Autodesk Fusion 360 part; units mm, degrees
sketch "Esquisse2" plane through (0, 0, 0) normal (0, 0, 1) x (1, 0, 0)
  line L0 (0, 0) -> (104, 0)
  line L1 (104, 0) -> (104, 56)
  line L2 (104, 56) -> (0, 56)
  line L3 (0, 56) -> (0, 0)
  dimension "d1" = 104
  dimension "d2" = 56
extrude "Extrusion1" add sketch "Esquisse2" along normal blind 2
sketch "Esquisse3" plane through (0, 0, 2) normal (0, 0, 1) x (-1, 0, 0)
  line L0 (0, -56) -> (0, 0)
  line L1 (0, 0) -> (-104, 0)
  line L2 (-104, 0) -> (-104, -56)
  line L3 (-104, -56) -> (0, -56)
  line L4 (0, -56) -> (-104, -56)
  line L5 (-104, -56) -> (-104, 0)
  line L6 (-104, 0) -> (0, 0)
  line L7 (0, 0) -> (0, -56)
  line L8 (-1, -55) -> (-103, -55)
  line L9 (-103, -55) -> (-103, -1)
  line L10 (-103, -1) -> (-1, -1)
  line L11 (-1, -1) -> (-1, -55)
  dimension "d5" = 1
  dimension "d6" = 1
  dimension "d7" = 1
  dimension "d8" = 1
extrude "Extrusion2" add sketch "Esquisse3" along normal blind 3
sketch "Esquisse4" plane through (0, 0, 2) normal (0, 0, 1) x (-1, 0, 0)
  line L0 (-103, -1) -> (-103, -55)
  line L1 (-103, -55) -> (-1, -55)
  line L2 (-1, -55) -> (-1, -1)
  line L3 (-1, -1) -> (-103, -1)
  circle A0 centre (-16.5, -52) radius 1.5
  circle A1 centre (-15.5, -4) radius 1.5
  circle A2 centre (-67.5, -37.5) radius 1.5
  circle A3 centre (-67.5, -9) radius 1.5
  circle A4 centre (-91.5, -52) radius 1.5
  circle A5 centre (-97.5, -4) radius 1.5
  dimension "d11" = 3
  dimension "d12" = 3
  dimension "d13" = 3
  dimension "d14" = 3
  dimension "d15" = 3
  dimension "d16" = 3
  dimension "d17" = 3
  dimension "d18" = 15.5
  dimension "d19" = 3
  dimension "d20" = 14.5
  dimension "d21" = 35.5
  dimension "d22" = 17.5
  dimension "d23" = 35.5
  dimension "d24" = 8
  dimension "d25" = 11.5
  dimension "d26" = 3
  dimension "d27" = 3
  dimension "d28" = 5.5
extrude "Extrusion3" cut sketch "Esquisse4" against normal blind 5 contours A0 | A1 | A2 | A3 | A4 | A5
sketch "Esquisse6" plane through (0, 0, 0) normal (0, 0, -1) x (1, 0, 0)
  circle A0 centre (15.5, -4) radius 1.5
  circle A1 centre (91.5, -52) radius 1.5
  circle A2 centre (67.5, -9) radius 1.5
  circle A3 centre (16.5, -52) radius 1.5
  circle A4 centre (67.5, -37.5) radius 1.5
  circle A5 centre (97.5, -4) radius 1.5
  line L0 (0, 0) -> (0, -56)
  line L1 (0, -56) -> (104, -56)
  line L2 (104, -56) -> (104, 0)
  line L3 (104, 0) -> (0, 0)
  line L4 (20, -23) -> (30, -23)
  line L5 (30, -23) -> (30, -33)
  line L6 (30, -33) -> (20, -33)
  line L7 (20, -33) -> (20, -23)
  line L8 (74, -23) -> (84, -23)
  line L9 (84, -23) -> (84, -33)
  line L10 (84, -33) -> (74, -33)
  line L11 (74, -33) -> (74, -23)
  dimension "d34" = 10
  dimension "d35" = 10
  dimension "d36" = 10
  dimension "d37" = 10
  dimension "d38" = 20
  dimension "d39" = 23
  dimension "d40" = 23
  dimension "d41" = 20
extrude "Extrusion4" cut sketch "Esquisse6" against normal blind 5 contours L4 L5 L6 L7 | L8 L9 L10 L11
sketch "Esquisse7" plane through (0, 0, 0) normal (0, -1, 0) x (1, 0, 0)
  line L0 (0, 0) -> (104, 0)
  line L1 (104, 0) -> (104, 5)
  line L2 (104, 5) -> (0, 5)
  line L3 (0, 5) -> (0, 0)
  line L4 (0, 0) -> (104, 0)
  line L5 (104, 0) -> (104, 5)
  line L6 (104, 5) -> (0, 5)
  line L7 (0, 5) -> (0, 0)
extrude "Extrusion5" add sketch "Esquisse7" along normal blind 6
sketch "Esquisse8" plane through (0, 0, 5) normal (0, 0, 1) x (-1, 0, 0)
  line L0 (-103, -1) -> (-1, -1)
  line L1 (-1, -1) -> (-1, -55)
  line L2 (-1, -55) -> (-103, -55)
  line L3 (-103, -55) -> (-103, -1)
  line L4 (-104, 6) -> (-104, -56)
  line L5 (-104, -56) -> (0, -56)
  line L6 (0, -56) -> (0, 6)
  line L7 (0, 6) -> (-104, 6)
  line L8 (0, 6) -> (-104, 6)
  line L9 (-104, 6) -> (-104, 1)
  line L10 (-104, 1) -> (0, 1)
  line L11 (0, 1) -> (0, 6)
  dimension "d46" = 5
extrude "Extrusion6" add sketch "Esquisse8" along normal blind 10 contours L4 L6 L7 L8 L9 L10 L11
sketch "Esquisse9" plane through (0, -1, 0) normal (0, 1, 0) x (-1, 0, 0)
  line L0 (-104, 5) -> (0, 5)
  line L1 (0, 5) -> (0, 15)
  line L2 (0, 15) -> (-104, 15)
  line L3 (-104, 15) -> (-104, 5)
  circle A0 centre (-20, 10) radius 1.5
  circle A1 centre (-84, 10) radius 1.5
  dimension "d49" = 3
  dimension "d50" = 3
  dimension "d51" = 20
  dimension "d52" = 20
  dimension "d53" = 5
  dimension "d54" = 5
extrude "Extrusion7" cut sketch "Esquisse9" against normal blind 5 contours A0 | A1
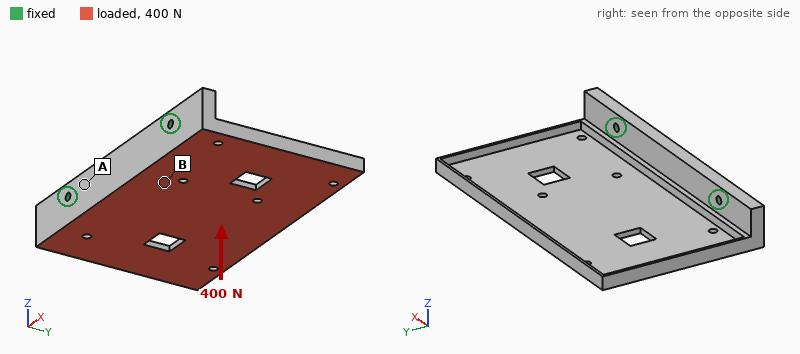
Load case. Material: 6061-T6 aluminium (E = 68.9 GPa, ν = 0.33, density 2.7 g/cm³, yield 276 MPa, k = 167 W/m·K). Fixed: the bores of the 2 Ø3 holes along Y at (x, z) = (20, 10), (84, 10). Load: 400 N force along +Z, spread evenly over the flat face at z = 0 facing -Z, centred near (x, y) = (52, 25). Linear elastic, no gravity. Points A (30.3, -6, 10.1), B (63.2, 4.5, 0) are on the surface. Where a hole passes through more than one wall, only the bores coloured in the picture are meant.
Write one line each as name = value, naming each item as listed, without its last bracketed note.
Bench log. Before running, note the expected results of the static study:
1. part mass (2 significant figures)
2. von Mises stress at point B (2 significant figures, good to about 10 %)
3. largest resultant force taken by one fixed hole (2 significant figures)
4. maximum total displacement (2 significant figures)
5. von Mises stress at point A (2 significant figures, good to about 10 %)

part mass = 55 g
von Mises stress at point B = 83 MPa
largest resultant force taken by one fixed hole = 200 N
maximum total displacement = 1.4 mm
von Mises stress at point A = 26 MPa
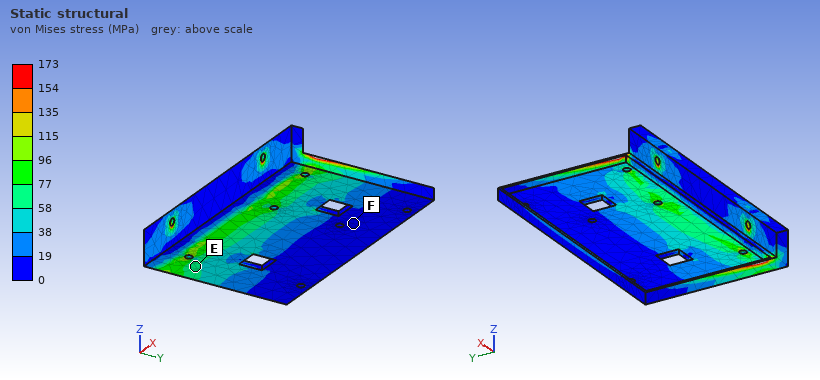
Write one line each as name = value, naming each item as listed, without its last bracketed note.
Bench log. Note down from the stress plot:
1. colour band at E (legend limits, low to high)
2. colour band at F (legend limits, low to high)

colour band at E = 58 to 77 MPa
colour band at F = 0 to 19 MPa
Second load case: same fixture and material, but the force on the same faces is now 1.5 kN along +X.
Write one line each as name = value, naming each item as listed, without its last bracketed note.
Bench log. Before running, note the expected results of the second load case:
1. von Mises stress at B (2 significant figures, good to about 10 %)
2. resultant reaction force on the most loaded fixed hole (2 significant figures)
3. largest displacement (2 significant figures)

von Mises stress at B = 11 MPa
resultant reaction force on the most loaded fixed hole = 1.0 kN
largest displacement = 56 µm
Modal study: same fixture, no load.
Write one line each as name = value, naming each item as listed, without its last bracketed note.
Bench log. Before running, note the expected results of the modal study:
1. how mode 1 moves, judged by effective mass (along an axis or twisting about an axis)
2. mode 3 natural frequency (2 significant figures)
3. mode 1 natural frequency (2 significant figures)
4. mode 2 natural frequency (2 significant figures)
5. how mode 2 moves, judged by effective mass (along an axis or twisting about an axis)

how mode 1 moves, judged by effective mass = along Z
mode 3 natural frequency = 2000 Hz
mode 1 natural frequency = 550 Hz
mode 2 natural frequency = 900 Hz
how mode 2 moves, judged by effective mass = twisting about Y
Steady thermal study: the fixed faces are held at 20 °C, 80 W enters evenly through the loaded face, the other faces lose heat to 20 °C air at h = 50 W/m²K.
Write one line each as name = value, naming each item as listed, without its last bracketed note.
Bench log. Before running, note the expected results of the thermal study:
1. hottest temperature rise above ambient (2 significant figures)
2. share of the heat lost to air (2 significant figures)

hottest temperature rise above ambient = 62 K
share of the heat lost to air = 26 %
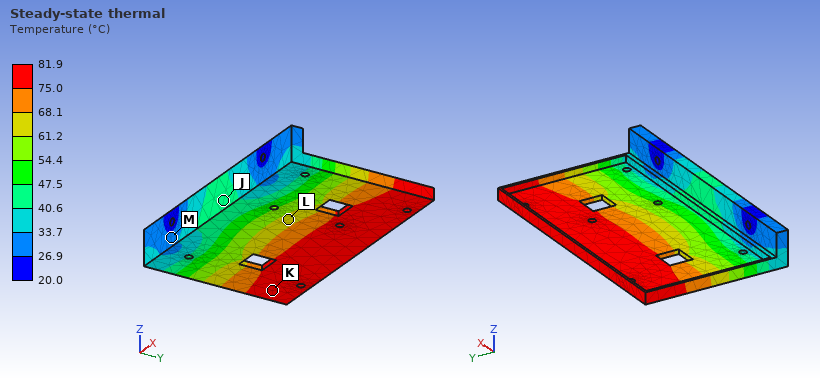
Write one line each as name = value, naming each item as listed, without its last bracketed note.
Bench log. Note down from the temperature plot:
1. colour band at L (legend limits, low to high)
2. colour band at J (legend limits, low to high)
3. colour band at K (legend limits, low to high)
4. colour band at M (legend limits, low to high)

colour band at L = 61.2 to 68.1 °C
colour band at J = 40.6 to 47.5 °C
colour band at K = 75.0 to 81.9 °C
colour band at M = 26.9 to 33.7 °C
